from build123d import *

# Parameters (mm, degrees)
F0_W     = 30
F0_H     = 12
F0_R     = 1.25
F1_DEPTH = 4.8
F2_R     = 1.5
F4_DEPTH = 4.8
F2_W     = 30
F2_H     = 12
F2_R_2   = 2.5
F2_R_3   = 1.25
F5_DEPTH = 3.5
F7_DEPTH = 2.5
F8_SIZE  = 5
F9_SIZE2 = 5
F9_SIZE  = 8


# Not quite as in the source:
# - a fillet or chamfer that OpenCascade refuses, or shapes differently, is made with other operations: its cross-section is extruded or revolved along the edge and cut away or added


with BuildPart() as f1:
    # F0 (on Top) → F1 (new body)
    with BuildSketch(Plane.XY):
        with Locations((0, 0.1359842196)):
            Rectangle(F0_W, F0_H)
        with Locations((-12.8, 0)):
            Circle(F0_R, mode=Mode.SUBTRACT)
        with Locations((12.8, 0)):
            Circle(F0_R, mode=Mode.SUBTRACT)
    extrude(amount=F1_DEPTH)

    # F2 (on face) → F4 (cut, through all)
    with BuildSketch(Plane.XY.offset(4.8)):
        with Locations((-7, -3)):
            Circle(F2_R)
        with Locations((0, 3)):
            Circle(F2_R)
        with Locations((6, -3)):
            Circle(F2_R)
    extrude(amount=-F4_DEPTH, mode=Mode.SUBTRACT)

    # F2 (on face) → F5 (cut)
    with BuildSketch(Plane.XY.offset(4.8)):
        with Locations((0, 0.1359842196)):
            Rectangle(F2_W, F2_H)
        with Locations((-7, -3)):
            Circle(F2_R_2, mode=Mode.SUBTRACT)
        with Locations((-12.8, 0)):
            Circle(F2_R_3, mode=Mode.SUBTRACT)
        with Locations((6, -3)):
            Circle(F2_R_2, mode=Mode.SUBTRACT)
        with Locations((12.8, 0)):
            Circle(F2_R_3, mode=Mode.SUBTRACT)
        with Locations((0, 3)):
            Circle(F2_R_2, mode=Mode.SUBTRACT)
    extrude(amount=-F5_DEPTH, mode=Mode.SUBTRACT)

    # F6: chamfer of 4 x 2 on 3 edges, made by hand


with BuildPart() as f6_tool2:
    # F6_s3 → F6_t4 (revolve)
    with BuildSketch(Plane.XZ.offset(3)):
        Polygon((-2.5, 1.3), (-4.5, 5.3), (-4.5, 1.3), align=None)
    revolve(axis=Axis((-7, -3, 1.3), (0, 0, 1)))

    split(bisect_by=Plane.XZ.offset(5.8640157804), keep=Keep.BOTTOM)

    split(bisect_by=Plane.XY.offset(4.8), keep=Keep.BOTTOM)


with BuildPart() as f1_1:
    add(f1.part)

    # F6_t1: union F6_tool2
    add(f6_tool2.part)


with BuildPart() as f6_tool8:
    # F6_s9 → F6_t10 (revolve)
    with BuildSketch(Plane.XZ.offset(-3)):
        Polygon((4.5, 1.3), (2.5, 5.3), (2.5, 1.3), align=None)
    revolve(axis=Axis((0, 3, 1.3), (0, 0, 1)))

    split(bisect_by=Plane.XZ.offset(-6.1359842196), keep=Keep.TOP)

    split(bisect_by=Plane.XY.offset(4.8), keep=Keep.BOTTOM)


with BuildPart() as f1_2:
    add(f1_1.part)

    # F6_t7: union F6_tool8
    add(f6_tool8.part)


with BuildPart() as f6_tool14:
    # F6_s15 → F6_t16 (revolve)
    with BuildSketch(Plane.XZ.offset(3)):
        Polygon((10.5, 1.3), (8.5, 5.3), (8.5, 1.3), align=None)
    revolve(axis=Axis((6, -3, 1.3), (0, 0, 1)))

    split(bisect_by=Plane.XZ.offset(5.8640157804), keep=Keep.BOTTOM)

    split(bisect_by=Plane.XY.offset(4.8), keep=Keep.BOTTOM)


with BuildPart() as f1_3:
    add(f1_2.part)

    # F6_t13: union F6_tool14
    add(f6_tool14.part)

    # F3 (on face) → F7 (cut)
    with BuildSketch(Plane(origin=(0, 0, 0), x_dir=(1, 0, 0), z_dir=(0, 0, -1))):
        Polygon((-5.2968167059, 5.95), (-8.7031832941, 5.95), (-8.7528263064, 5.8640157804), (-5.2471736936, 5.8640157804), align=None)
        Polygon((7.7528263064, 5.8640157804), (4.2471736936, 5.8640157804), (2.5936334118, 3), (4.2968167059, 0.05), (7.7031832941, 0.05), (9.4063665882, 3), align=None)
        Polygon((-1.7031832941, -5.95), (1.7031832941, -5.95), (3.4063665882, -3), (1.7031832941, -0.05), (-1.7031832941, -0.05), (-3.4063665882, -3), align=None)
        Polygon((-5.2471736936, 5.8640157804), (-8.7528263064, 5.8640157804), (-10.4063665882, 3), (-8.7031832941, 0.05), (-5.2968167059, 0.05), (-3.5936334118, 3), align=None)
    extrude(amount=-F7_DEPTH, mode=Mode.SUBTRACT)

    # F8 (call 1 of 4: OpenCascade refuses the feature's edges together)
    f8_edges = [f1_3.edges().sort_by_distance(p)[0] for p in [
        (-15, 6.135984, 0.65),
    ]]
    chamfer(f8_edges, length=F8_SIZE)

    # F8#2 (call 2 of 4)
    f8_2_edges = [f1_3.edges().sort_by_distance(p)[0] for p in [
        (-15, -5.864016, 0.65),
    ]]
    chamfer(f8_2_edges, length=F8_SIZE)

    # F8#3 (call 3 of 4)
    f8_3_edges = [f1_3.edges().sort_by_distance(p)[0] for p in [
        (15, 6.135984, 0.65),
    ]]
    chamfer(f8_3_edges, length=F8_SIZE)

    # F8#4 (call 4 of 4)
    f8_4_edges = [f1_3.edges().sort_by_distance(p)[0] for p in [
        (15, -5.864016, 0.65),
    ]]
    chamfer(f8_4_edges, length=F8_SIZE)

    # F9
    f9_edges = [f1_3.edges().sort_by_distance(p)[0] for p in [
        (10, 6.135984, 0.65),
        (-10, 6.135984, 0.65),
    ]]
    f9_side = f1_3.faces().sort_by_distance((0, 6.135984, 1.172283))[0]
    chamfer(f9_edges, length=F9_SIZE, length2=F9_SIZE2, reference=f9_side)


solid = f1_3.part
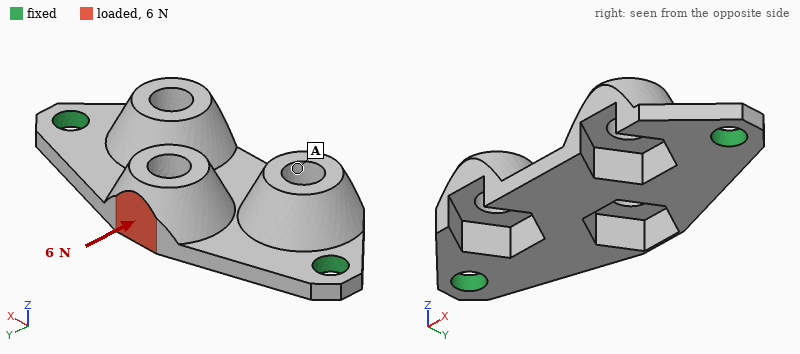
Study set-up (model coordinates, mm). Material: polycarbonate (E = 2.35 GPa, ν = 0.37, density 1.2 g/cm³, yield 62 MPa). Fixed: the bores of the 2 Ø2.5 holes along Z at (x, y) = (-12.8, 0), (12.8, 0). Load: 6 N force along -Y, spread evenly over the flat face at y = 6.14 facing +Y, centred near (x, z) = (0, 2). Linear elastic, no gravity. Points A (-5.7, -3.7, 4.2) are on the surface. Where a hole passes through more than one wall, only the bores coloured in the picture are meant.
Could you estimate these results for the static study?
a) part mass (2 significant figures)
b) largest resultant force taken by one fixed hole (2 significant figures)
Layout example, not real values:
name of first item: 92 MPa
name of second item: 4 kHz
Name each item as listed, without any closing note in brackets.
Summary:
part mass: 0.59 g
largest resultant force taken by one fixed hole: 3.3 N
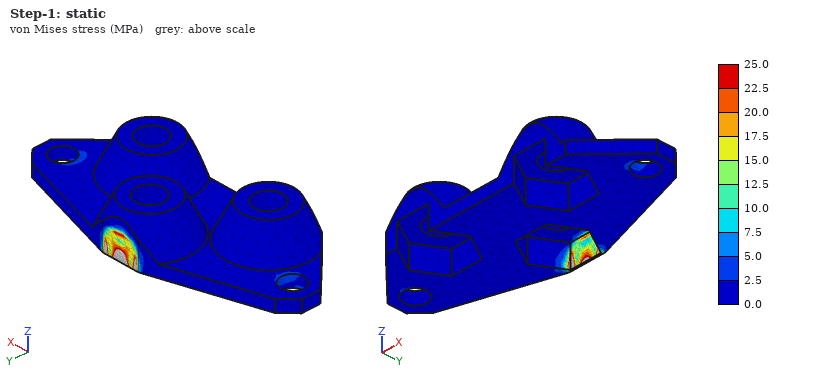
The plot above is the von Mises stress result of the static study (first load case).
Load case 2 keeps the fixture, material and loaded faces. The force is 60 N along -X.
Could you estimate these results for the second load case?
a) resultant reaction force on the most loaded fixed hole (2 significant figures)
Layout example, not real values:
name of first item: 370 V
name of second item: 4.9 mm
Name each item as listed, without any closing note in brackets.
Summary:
resultant reaction force on the most loaded fixed hole: 34 N
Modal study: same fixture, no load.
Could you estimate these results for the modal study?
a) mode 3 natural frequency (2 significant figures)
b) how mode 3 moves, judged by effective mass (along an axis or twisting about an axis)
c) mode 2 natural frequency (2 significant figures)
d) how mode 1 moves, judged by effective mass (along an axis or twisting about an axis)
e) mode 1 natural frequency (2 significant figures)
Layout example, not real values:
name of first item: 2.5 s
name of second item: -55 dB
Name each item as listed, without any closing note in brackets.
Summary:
mode 3 natural frequency: 6200 Hz
how mode 3 moves, judged by effective mass: along Y
mode 2 natural frequency: 3400 Hz
how mode 1 moves, judged by effective mass: along Z
mode 1 natural frequency: 2800 Hz
